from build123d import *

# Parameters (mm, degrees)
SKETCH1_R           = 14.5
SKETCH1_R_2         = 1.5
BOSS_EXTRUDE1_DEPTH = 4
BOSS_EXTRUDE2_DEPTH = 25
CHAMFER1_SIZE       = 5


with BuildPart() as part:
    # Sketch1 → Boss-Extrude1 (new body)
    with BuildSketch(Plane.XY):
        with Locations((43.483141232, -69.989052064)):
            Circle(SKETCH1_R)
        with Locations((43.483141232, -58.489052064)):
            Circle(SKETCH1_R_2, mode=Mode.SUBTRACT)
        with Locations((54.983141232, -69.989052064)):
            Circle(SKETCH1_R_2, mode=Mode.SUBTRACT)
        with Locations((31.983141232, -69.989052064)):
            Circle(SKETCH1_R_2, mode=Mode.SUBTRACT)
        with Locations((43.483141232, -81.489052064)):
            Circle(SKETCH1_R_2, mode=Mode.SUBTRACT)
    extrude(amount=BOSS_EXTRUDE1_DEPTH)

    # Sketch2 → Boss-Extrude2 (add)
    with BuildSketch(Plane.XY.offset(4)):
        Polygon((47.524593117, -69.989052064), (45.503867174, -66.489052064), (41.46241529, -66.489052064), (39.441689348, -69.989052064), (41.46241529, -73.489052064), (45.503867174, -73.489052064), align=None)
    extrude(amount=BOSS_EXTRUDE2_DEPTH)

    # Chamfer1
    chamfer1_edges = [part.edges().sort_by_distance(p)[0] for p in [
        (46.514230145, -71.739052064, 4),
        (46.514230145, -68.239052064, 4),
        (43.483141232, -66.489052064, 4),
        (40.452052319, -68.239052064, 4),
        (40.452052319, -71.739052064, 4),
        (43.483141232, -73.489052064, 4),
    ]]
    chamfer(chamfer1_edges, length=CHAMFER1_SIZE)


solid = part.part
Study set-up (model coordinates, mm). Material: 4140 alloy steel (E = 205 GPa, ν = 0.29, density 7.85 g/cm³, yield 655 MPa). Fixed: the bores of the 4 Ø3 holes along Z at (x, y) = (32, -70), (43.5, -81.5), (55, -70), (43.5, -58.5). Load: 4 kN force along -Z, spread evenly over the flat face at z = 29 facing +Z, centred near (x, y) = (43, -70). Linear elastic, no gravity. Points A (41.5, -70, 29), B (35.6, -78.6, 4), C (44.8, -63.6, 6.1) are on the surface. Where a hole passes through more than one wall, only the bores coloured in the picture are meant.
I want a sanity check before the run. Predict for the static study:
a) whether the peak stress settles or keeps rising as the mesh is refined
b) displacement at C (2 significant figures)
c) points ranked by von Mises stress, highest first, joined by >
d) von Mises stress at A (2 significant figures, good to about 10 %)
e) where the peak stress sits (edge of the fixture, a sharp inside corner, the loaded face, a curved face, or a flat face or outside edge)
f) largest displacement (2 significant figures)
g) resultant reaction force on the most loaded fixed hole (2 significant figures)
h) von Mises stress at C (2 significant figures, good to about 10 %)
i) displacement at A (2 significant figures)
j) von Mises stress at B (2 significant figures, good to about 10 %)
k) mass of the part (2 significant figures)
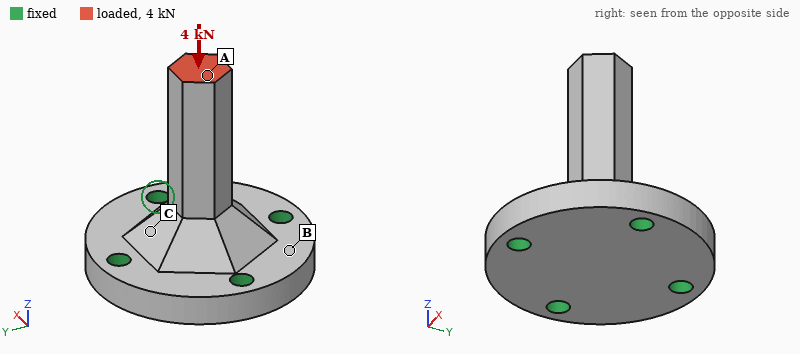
keeps rising
2.6 µm
A > C > B
94 MPa
edge of the fixture
14 µm
1.1 kN
51 MPa
14 µm
19 MPa
32 g
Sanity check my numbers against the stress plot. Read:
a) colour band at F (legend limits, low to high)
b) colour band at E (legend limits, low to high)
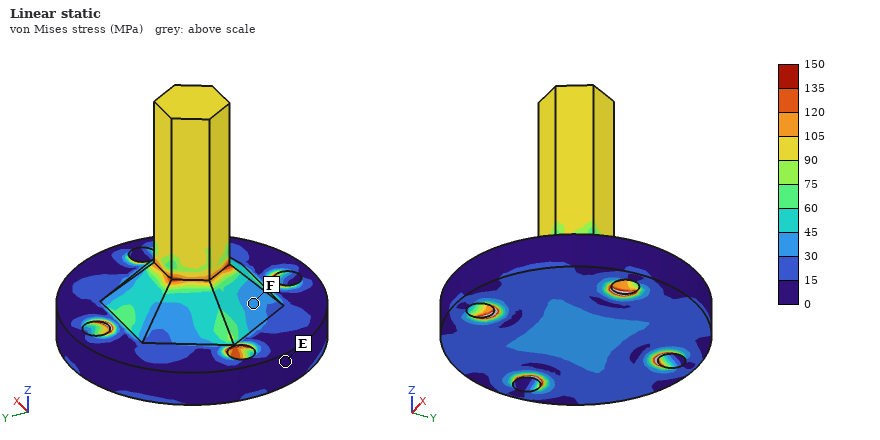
30 to 45 MPa
0 to 15 MPa
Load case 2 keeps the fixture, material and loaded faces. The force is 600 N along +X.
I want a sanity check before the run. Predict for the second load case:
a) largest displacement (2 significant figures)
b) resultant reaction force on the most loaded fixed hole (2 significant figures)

82 µm
800 N
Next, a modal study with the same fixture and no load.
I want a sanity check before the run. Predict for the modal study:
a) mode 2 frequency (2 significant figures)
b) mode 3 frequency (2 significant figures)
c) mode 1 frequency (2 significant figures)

9900 Hz
36 kHz
9900 Hz
